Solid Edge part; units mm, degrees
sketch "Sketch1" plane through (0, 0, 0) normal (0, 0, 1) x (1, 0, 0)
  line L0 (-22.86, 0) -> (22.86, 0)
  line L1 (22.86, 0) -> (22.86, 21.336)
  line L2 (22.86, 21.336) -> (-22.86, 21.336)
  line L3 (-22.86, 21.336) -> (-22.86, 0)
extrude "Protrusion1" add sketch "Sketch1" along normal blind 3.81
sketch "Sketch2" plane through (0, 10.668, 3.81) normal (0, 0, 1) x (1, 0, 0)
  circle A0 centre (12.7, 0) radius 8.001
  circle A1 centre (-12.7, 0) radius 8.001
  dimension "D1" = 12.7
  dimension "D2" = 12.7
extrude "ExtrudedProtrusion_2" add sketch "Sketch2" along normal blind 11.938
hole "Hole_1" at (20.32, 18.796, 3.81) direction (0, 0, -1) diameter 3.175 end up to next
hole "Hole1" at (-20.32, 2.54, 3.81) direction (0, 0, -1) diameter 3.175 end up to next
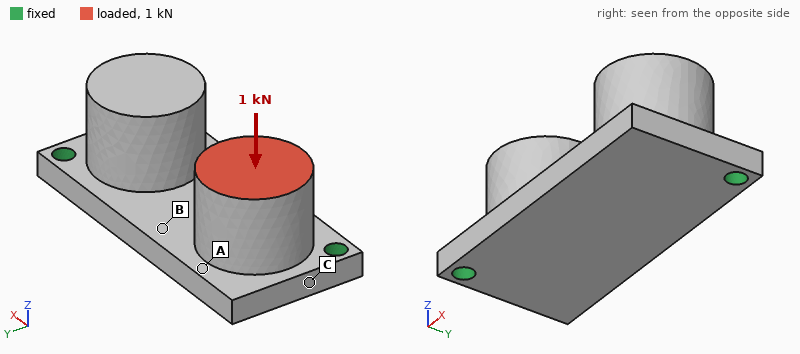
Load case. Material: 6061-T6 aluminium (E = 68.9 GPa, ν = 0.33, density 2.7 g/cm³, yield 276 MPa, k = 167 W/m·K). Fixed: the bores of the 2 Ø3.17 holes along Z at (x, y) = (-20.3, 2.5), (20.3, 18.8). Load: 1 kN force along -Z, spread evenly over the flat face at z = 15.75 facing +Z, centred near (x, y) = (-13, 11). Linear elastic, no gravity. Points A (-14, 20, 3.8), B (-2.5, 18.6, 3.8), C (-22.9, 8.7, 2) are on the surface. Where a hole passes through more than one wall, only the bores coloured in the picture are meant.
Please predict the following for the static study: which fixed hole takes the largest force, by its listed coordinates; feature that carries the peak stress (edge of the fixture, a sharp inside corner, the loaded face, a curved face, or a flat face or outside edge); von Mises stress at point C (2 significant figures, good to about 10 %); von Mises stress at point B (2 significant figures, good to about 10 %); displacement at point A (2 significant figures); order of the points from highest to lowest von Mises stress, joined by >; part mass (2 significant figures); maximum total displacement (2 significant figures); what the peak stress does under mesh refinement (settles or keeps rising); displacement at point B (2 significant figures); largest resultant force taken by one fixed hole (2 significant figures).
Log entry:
(-20.3, 2.5)
edge of the fixture
32 MPa
48 MPa
69 µm
B > C > A
23 g
85 µm
keeps rising
63 µm
800 N
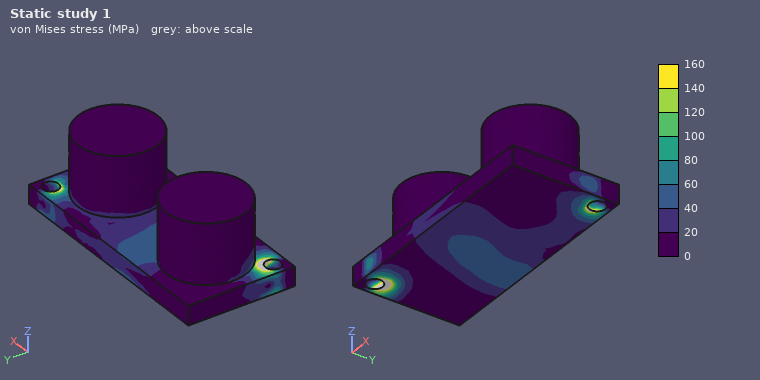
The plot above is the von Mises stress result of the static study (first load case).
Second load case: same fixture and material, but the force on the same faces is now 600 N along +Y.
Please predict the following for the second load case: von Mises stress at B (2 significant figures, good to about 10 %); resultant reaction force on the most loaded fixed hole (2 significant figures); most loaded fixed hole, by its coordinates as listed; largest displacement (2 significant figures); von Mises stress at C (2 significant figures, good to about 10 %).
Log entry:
32 MPa
510 N
(-20.3, 2.5)
0.11 mm
66 MPa
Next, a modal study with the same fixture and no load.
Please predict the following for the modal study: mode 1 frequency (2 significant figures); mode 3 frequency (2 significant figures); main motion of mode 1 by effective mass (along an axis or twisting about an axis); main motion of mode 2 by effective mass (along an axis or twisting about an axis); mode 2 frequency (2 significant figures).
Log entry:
4900 Hz
8800 Hz
along Y
along Z
5200 Hz
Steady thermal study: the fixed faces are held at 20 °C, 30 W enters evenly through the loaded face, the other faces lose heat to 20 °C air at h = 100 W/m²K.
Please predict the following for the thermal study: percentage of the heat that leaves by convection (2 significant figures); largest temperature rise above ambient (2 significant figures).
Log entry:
13 %
28 K
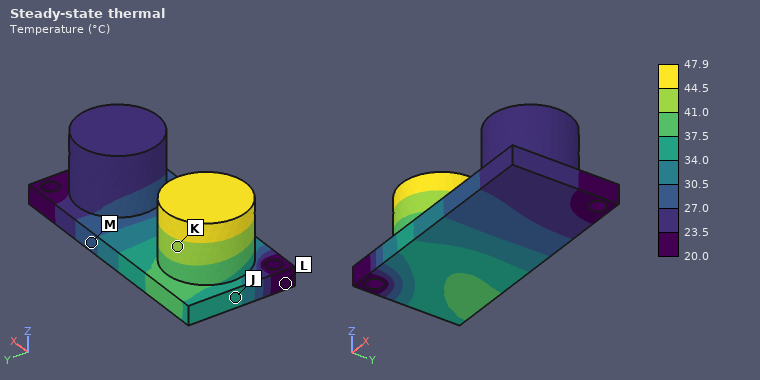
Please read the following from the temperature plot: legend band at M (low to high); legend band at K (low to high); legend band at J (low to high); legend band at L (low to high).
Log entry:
27.0 to 30.5 °C
41.0 to 44.5 °C
34.0 to 37.5 °C
20.0 to 23.5 °C
